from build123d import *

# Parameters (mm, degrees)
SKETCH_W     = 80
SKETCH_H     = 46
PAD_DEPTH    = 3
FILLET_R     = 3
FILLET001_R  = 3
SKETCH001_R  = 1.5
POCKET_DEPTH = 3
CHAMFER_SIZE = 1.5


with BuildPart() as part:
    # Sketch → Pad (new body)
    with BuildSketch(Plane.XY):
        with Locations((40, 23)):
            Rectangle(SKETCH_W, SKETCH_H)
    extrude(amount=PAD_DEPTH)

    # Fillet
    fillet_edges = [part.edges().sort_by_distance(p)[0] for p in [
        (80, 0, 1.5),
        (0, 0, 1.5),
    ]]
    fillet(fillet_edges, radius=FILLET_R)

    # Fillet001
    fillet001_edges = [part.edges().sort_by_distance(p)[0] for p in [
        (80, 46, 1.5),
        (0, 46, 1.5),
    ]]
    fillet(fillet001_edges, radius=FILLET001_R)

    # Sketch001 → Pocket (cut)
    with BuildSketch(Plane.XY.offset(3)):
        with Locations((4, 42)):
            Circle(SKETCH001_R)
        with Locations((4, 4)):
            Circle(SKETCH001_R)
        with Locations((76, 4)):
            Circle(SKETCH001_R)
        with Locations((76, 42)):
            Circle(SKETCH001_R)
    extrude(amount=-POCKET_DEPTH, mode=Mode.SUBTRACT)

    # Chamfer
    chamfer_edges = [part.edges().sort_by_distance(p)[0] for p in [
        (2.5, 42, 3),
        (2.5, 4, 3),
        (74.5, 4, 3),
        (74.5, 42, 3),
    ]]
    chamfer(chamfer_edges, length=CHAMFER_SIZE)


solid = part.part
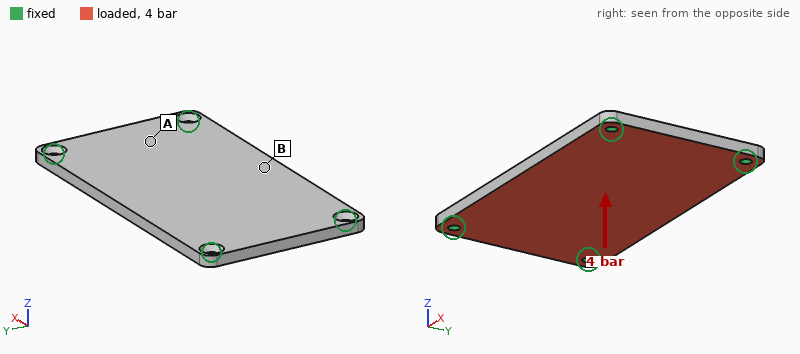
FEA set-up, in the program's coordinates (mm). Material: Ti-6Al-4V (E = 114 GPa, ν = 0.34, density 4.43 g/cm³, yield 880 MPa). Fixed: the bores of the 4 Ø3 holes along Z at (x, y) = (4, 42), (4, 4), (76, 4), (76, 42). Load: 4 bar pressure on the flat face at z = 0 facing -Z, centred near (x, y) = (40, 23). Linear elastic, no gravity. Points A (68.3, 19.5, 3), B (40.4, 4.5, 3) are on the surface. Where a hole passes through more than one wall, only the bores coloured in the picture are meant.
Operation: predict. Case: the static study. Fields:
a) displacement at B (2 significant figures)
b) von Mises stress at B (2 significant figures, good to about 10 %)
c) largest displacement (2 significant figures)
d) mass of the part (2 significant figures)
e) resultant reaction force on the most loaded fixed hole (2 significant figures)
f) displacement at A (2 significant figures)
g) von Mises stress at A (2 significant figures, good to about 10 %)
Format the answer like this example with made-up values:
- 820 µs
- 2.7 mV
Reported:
- 0.19 mm
- 86 MPa
- 0.19 mm
- 48 g
- 590 N
- 0.064 mm
- 32 MPa
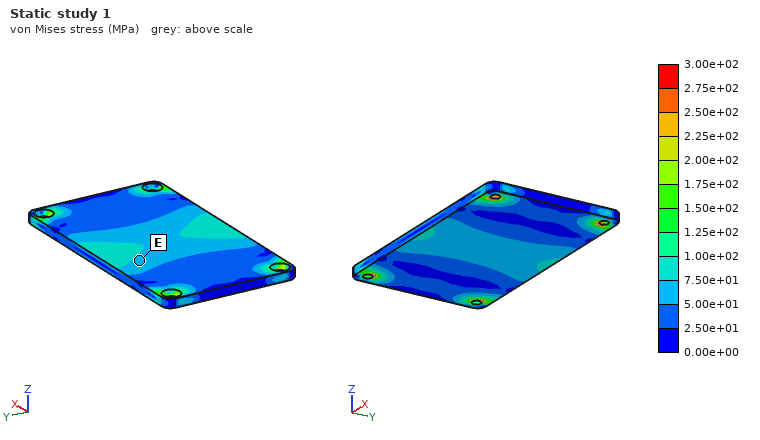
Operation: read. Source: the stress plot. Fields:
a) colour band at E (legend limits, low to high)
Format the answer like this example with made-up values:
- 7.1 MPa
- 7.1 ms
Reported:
- 5.00e+01 to 7.50e+01 MPa
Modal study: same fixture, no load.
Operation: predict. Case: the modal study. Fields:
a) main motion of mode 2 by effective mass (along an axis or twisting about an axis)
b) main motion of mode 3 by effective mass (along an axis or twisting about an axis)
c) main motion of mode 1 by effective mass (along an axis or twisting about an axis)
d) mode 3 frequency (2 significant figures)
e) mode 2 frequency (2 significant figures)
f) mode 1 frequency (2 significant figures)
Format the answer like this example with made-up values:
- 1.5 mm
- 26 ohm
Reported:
- twisting about X
- twisting about Y
- along Z
- 6300 Hz
- 4000 Hz
- 2300 Hz
